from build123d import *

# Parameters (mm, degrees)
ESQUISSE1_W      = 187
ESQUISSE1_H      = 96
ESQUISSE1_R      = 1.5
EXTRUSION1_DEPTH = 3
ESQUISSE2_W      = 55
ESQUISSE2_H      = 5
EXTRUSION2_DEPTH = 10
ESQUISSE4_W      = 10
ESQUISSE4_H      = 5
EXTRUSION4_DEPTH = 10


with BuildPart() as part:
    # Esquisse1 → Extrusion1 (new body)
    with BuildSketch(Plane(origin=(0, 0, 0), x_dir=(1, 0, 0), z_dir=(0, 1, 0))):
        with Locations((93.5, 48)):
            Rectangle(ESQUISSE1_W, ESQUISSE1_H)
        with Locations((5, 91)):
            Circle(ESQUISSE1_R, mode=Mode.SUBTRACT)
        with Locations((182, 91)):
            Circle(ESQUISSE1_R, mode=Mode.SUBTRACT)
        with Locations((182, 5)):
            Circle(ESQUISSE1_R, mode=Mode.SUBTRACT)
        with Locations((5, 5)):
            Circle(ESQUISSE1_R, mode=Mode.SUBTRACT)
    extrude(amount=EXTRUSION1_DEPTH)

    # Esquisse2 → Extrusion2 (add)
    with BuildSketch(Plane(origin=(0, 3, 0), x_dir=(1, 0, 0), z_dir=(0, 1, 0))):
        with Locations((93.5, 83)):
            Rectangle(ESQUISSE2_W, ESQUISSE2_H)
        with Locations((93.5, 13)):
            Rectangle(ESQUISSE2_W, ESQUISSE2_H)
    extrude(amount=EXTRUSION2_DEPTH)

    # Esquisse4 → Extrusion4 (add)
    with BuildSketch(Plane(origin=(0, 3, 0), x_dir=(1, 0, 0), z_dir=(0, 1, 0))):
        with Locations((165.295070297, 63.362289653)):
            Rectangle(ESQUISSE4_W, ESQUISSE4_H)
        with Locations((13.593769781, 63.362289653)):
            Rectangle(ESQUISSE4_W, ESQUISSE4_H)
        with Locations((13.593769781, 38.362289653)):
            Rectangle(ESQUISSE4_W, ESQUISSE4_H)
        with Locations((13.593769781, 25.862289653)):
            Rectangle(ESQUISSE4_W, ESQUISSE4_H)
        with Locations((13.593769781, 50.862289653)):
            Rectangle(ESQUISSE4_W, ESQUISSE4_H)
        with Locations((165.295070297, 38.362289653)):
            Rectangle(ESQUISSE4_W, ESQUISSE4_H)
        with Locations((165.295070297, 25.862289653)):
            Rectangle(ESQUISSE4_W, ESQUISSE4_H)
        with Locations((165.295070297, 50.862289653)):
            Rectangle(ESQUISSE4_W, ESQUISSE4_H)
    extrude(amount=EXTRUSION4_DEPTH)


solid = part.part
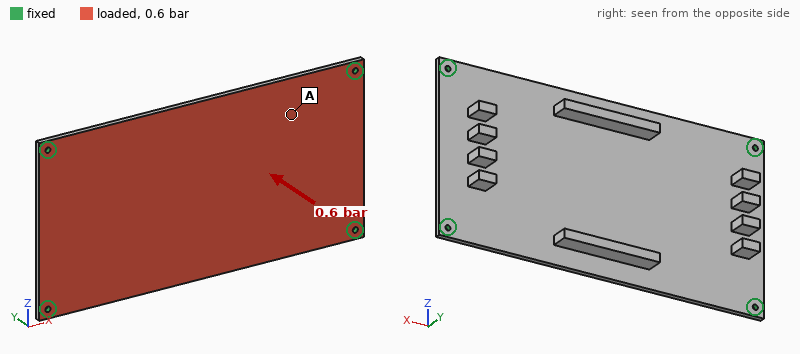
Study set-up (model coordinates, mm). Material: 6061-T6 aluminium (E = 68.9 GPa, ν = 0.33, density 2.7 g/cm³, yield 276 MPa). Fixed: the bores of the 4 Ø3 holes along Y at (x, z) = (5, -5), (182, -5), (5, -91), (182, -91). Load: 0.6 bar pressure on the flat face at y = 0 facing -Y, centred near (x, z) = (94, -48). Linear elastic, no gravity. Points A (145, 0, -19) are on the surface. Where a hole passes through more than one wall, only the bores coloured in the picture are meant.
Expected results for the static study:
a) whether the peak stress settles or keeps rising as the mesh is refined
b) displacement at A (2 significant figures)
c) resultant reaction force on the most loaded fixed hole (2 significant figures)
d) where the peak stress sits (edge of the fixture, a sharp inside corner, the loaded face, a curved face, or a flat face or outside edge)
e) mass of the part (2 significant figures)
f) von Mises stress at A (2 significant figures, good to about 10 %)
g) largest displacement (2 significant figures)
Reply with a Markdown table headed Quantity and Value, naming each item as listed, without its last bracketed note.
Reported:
| Quantity | Value |
|---|---|
| whether the peak stress settles or keeps rising as the mesh is refined | keeps rising |
| displacement at A | 0.61 mm |
| resultant reaction force on the most loaded fixed hole | 290 N |
| where the peak stress sits | edge of the fixture |
| mass of the part | 170 g |
| von Mises stress at A | 32 MPa |
| largest displacement | 0.96 mm |
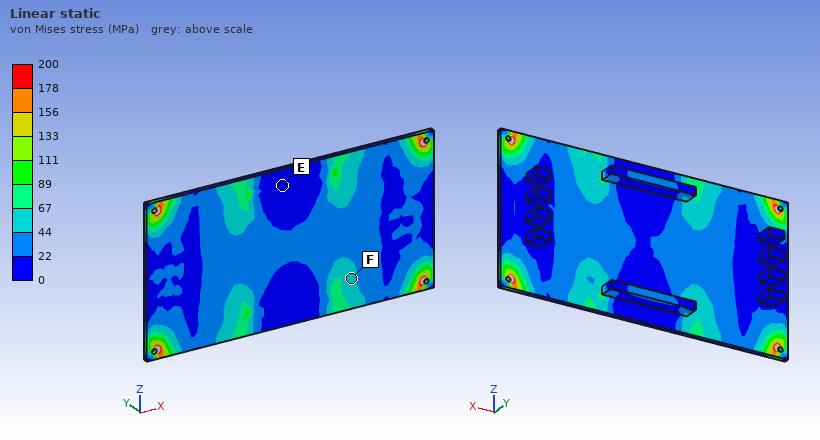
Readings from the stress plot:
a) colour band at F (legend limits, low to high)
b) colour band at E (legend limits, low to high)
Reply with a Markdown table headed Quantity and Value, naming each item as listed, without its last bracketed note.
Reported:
| Quantity | Value |
|---|---|
| colour band at F | 44 to 67 MPa |
| colour band at E | 0 to 22 MPa |
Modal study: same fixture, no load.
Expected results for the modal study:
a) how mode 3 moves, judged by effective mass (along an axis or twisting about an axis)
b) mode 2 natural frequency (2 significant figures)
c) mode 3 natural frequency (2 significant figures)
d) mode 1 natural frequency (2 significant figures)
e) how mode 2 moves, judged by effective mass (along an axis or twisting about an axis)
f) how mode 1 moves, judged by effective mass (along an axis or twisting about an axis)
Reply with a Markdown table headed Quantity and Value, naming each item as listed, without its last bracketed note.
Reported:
| Quantity | Value |
|---|---|
| how mode 3 moves, judged by effective mass | twisting about Z |
| mode 2 natural frequency | 760 Hz |
| mode 3 natural frequency | 1100 Hz |
| mode 1 natural frequency | 450 Hz |
| how mode 2 moves, judged by effective mass | twisting about X |
| how mode 1 moves, judged by effective mass | along Y |
